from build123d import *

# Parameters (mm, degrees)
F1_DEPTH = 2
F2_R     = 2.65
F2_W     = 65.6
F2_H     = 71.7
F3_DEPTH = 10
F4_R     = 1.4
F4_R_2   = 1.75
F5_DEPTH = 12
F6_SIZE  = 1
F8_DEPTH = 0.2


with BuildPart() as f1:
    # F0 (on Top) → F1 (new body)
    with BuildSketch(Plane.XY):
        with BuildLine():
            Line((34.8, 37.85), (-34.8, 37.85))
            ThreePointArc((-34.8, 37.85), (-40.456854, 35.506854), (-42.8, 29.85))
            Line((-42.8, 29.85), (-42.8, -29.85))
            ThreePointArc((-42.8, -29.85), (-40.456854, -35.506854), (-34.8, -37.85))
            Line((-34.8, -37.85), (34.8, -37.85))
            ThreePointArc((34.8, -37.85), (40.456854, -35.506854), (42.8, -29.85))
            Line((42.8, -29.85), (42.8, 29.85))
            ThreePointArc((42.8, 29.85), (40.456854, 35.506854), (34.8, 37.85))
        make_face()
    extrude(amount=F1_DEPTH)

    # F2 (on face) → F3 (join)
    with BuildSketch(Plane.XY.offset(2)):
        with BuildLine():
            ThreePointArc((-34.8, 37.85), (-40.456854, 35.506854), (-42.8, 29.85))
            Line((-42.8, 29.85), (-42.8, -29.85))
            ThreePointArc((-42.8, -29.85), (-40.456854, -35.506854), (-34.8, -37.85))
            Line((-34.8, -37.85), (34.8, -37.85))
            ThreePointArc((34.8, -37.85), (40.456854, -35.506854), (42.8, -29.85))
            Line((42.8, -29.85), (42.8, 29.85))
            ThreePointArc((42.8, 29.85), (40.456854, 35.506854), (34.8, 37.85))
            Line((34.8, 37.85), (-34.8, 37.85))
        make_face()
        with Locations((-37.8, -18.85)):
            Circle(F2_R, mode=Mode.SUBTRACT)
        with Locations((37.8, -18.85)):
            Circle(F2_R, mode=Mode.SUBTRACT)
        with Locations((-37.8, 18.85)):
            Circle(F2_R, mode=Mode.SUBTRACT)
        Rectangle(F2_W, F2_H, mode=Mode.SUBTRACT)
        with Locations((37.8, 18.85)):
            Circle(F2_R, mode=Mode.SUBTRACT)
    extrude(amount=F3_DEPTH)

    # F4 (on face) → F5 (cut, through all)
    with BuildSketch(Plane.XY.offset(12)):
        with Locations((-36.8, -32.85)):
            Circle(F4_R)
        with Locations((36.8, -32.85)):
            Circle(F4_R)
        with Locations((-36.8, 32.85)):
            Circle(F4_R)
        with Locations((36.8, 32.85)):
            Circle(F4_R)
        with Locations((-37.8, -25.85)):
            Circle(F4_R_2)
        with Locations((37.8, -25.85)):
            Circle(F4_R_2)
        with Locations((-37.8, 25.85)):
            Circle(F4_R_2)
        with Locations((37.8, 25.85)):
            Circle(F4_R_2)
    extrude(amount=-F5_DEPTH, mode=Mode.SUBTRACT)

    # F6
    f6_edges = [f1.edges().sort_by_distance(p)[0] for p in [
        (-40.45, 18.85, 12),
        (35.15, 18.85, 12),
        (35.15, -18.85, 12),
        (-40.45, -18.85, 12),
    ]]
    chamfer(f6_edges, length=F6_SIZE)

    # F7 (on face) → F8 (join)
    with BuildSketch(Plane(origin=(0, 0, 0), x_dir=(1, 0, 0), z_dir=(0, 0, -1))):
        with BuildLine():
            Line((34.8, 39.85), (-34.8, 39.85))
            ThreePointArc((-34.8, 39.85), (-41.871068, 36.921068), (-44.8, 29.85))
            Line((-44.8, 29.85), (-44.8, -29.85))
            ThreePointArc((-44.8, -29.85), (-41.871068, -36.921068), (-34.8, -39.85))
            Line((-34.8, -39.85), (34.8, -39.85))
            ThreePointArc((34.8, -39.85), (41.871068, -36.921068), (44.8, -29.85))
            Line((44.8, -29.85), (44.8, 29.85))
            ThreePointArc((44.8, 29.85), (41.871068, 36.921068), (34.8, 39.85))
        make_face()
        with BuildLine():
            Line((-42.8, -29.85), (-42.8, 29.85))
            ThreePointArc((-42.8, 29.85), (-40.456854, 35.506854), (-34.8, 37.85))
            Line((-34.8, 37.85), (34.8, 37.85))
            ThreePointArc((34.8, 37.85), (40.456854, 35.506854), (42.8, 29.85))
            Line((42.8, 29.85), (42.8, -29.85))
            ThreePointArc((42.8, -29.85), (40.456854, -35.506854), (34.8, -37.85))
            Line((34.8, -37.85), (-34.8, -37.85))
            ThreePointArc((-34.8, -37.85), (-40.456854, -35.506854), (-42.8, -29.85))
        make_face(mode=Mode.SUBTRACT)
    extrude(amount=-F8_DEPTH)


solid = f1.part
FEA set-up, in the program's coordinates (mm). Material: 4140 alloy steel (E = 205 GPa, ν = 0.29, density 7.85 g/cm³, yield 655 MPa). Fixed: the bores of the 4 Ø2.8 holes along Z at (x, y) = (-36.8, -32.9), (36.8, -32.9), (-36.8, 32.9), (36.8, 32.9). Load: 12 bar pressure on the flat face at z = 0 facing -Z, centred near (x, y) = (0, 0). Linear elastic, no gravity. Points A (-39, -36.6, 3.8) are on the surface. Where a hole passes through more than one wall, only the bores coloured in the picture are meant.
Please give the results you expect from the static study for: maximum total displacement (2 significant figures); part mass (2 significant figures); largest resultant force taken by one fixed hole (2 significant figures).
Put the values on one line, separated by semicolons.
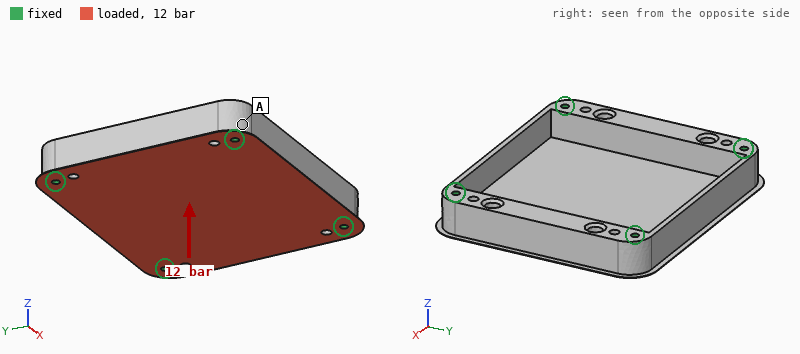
0.35 mm; 220 g; 2.3 kN
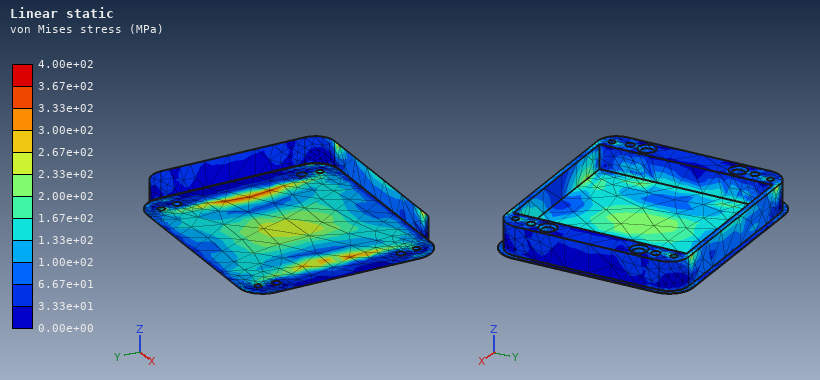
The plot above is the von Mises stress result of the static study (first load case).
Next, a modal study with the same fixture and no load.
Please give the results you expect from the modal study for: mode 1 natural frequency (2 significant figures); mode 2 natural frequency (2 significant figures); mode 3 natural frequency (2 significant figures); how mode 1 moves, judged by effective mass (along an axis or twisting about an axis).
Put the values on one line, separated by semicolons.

2900 Hz; 5000 Hz; 6700 Hz; along Z
